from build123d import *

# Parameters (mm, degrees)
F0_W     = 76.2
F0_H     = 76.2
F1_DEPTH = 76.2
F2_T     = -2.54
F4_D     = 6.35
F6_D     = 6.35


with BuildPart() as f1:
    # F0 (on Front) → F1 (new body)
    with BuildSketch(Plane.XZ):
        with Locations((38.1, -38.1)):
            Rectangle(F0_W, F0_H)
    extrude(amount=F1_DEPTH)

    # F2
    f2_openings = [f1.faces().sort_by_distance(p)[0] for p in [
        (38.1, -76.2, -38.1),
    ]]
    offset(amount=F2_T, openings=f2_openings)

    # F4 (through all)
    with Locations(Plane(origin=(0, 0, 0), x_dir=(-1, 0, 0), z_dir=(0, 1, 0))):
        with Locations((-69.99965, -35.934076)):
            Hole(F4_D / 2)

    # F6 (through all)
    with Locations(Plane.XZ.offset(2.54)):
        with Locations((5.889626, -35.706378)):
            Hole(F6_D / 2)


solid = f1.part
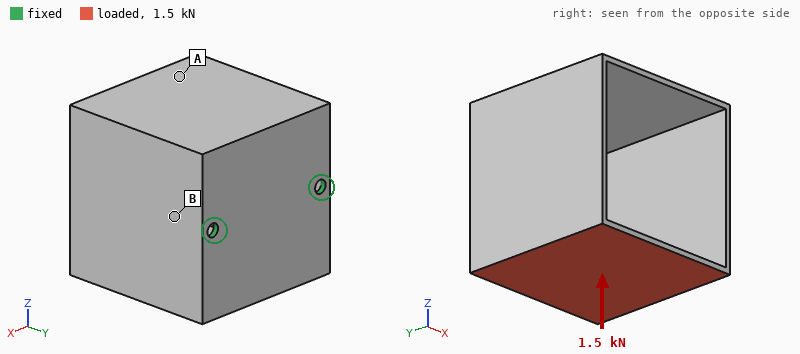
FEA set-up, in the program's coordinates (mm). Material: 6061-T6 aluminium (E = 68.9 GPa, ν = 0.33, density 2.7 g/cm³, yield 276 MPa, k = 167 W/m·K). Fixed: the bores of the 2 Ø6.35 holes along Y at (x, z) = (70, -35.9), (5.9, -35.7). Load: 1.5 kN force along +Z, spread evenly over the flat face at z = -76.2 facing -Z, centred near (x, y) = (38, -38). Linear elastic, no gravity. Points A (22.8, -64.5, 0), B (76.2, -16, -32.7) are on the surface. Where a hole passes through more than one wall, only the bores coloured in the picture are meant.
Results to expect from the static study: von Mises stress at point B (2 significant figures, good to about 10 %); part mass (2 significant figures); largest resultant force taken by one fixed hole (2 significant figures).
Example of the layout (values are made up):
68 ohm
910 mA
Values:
53 MPa
190 g
770 N
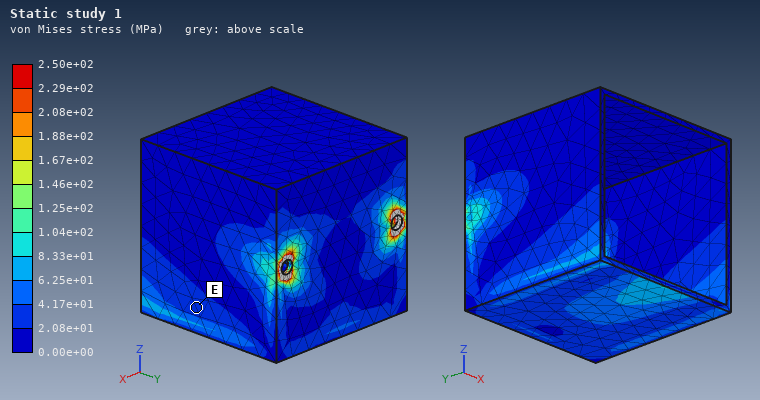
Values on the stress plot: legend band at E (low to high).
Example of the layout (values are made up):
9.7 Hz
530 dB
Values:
2.08e+01 to 4.17e+01 MPa
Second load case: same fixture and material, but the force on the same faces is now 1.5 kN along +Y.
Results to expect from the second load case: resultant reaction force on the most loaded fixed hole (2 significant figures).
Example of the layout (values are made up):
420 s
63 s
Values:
750 N
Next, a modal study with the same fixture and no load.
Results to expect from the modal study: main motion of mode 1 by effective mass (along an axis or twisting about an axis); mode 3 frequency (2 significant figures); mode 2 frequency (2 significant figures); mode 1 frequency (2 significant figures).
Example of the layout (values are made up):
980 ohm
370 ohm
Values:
along Z
1400 Hz
850 Hz
490 Hz
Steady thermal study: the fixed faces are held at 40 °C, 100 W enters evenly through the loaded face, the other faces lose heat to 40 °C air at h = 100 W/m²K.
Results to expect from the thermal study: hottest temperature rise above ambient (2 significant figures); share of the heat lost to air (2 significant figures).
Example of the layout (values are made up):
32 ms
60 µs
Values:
52 K
74 %
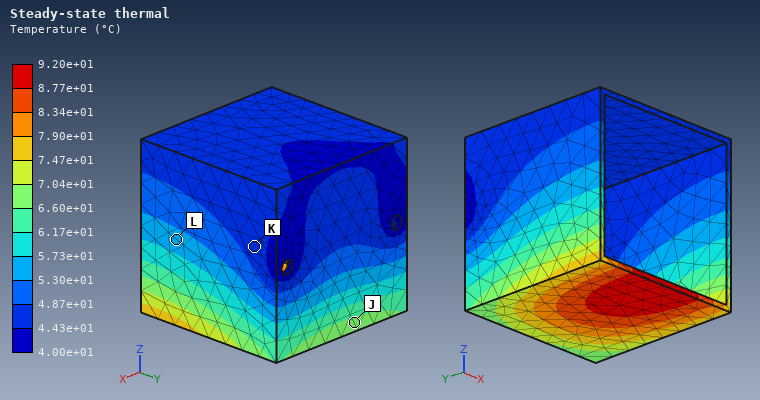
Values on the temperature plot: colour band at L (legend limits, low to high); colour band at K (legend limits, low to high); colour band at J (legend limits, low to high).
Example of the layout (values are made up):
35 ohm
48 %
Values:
5.30e+01 to 5.73e+01 °C
4.43e+01 to 4.87e+01 °C
6.60e+01 to 7.04e+01 °C
